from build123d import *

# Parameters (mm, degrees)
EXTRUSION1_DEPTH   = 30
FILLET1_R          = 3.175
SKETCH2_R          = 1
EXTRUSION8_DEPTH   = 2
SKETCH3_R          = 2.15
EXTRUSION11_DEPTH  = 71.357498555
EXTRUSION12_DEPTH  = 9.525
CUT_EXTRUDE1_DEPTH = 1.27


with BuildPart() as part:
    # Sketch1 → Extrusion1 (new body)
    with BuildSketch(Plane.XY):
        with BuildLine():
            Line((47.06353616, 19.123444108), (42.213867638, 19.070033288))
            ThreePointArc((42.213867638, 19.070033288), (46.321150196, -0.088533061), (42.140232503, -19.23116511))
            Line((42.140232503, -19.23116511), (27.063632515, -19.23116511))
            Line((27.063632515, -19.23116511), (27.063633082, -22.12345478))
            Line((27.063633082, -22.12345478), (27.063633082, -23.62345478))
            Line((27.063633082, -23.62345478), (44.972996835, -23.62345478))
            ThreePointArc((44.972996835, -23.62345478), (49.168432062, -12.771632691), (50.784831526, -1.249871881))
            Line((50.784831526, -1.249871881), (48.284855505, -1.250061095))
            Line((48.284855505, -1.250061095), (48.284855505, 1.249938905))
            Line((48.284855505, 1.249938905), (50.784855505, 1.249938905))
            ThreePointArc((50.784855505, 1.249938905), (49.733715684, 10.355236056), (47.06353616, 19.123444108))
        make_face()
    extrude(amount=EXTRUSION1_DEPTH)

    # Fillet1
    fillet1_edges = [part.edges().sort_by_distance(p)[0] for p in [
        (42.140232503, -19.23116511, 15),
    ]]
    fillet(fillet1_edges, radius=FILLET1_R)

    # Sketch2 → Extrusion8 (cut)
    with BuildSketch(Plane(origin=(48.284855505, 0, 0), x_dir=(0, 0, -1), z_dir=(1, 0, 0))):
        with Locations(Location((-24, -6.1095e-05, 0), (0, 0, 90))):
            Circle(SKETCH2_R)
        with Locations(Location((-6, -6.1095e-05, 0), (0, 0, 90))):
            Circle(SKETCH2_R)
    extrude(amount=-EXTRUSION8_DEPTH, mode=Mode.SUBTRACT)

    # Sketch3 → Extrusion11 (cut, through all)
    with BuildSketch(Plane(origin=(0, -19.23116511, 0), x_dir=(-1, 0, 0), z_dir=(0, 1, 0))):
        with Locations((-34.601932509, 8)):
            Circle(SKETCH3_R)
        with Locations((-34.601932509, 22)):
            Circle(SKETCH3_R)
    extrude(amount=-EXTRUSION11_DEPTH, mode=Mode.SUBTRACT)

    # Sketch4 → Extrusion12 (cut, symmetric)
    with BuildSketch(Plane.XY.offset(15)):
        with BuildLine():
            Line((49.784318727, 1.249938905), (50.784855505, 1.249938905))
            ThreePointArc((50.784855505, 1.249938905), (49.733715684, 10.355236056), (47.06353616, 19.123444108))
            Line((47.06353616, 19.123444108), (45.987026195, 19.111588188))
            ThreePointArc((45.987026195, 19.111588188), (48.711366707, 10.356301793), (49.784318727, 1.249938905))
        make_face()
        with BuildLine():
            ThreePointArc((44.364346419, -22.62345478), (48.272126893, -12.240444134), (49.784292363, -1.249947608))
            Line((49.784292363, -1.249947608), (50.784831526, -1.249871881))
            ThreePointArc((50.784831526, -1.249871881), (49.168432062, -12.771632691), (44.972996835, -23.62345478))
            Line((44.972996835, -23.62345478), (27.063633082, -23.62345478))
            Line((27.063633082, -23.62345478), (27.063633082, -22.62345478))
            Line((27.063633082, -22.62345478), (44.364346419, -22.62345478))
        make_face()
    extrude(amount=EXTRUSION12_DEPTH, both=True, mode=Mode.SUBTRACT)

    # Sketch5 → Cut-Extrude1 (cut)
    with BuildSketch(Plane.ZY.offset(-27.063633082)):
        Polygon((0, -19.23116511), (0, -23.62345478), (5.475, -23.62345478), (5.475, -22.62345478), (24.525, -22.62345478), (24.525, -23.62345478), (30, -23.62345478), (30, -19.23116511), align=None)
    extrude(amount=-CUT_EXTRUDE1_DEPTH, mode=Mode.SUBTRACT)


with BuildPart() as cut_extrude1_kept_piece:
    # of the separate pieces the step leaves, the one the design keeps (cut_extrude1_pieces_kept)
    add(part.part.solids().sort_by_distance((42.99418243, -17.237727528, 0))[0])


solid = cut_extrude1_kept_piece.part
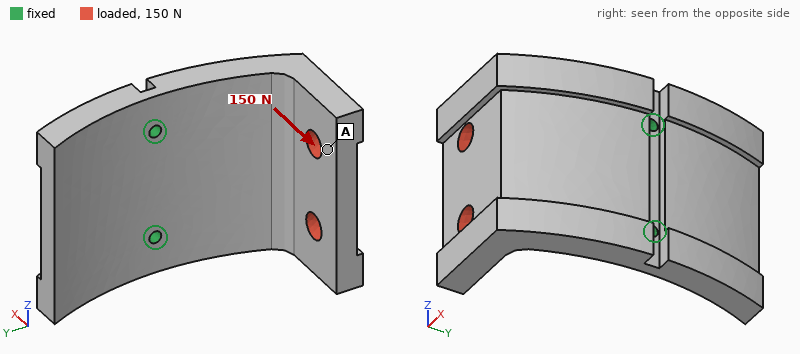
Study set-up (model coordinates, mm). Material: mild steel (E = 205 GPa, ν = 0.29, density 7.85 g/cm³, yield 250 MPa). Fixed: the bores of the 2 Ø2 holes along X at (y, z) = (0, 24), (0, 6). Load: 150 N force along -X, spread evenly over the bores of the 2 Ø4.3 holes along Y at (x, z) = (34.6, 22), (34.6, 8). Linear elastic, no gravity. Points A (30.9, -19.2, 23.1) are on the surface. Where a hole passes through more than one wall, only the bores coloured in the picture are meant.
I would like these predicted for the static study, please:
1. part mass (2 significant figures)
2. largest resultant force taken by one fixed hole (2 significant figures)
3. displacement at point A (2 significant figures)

49 g
81 N
65 µm
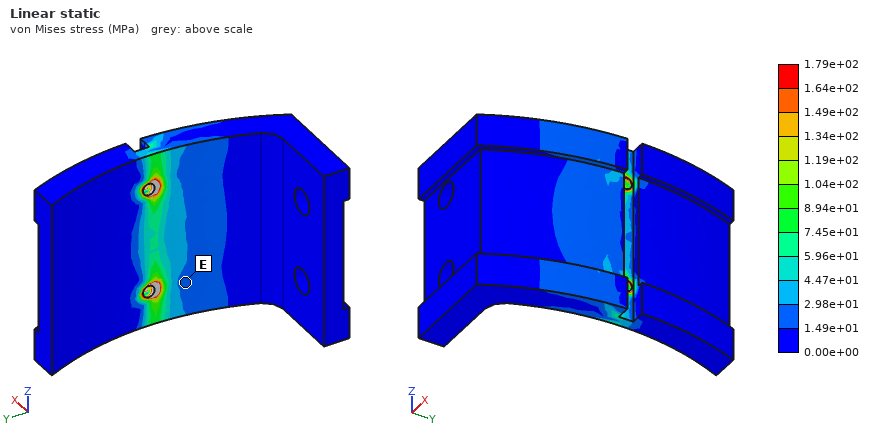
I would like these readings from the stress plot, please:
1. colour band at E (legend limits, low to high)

1.49e+01 to 2.98e+01 MPa
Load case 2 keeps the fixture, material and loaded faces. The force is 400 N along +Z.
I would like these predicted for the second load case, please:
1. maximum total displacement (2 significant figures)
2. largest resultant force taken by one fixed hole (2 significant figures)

46 µm
550 N
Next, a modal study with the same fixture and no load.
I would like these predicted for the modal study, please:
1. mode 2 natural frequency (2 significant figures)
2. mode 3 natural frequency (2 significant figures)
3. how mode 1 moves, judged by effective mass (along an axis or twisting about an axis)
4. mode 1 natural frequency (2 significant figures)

4200 Hz
4300 Hz
along X
1700 Hz
